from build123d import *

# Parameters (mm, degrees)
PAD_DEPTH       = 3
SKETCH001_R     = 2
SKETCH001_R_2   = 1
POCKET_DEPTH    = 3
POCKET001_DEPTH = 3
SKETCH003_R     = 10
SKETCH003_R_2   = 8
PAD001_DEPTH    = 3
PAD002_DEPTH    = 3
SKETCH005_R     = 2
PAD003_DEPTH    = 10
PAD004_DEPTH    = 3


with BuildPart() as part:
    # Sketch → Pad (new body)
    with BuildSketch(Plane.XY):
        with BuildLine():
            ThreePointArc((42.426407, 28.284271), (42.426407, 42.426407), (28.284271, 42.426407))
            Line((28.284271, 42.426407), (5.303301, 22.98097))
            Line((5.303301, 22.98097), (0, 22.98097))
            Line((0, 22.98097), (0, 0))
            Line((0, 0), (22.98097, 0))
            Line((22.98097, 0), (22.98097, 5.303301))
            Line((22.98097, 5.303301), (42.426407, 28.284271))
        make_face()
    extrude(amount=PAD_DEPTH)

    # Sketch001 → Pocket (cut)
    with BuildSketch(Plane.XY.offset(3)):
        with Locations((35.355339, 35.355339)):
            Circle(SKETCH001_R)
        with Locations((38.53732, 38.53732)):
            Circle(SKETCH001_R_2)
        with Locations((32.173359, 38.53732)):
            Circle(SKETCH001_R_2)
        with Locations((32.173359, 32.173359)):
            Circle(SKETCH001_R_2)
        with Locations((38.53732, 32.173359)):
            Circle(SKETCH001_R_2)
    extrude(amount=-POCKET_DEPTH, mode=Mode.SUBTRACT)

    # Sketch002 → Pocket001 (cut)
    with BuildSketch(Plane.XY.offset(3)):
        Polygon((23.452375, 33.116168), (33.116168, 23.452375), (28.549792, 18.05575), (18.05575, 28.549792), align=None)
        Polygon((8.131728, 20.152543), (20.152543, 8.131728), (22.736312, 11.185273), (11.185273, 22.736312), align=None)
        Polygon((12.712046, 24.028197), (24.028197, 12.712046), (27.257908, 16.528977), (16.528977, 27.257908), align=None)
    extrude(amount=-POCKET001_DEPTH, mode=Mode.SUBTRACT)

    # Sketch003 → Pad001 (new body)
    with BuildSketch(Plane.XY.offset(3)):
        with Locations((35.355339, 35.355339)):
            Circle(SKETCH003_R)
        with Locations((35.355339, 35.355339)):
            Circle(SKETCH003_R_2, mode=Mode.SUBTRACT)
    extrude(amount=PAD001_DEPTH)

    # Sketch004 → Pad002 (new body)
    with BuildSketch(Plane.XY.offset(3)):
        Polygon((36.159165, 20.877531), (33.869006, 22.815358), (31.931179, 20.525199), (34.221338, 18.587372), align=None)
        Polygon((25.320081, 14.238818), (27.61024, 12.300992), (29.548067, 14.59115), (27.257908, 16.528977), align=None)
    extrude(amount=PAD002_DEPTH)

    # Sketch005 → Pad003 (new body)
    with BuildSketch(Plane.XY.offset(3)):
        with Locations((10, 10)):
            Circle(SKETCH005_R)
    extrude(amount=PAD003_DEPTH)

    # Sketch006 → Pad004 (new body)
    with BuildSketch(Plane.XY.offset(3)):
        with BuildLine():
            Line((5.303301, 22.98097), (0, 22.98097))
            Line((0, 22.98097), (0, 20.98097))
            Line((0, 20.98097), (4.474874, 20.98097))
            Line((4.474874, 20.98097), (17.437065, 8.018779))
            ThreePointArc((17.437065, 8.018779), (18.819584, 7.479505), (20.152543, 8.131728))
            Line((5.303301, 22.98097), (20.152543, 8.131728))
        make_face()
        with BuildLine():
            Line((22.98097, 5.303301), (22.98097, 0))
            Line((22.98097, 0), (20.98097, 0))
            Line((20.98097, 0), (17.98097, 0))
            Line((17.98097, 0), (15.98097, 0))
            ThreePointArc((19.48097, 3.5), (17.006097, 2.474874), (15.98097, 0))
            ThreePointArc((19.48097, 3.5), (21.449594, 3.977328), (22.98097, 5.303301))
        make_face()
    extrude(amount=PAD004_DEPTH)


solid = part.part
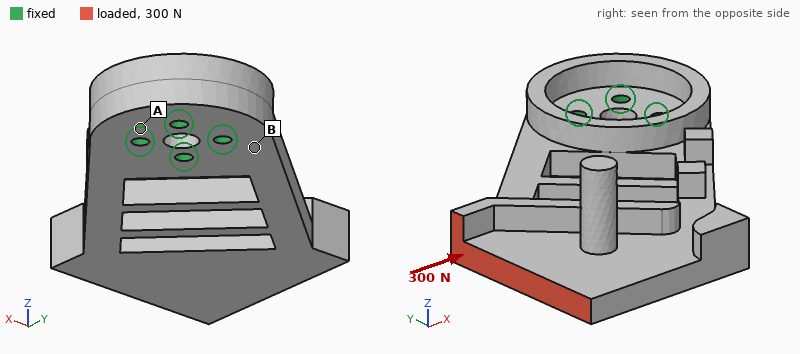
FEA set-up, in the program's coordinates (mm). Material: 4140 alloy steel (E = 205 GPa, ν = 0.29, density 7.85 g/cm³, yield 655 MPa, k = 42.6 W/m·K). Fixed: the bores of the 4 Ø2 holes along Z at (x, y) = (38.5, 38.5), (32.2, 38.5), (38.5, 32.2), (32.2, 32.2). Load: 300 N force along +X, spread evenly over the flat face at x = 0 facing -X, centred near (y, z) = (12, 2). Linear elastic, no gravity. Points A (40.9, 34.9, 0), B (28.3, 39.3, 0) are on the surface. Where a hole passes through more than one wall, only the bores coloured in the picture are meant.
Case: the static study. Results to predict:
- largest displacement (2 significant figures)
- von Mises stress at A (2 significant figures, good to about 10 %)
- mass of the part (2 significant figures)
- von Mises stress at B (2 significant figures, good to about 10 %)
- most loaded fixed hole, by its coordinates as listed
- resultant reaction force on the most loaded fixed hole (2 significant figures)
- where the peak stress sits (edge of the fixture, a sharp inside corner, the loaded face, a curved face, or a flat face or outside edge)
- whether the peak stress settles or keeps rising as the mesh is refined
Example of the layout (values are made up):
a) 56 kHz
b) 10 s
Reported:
a) 52 µm
b) 11 MPa
c) 28 g
d) 22 MPa
e) (32.2, 32.2)
f) 500 N
g) a sharp inside corner
h) keeps rising
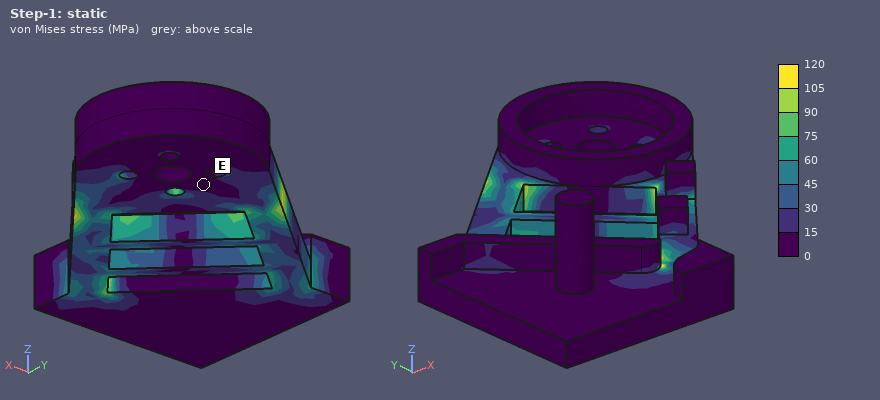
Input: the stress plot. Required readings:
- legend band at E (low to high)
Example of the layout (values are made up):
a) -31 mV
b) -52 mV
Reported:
a) 0 to 15 MPa
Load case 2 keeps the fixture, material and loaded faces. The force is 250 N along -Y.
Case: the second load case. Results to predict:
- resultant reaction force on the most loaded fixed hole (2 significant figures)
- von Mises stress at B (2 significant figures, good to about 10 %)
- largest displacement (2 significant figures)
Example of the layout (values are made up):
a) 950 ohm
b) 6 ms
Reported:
a) 560 N
b) 37 MPa
c) 57 µm
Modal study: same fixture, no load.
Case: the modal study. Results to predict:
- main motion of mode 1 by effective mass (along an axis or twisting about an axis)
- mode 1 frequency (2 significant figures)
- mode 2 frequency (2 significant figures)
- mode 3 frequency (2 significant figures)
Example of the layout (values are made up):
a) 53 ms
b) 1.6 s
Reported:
a) along Z
b) 900 Hz
c) 2800 Hz
d) 3200 Hz
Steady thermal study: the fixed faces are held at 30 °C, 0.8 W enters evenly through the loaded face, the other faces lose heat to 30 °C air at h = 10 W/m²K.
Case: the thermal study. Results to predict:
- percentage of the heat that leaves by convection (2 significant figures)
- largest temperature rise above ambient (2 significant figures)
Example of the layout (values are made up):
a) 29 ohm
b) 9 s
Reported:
a) 33 %
b) 17 K
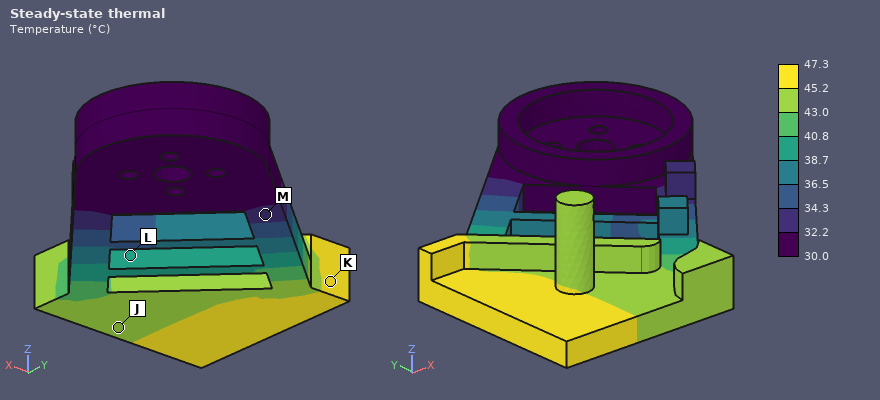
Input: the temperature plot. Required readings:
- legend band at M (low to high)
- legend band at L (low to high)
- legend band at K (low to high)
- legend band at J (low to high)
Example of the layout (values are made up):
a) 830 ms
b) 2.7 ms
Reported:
a) 32.2 to 34.3 °C
b) 38.7 to 40.8 °C
c) 45.2 to 47.3 °C
d) 43.0 to 45.2 °C
